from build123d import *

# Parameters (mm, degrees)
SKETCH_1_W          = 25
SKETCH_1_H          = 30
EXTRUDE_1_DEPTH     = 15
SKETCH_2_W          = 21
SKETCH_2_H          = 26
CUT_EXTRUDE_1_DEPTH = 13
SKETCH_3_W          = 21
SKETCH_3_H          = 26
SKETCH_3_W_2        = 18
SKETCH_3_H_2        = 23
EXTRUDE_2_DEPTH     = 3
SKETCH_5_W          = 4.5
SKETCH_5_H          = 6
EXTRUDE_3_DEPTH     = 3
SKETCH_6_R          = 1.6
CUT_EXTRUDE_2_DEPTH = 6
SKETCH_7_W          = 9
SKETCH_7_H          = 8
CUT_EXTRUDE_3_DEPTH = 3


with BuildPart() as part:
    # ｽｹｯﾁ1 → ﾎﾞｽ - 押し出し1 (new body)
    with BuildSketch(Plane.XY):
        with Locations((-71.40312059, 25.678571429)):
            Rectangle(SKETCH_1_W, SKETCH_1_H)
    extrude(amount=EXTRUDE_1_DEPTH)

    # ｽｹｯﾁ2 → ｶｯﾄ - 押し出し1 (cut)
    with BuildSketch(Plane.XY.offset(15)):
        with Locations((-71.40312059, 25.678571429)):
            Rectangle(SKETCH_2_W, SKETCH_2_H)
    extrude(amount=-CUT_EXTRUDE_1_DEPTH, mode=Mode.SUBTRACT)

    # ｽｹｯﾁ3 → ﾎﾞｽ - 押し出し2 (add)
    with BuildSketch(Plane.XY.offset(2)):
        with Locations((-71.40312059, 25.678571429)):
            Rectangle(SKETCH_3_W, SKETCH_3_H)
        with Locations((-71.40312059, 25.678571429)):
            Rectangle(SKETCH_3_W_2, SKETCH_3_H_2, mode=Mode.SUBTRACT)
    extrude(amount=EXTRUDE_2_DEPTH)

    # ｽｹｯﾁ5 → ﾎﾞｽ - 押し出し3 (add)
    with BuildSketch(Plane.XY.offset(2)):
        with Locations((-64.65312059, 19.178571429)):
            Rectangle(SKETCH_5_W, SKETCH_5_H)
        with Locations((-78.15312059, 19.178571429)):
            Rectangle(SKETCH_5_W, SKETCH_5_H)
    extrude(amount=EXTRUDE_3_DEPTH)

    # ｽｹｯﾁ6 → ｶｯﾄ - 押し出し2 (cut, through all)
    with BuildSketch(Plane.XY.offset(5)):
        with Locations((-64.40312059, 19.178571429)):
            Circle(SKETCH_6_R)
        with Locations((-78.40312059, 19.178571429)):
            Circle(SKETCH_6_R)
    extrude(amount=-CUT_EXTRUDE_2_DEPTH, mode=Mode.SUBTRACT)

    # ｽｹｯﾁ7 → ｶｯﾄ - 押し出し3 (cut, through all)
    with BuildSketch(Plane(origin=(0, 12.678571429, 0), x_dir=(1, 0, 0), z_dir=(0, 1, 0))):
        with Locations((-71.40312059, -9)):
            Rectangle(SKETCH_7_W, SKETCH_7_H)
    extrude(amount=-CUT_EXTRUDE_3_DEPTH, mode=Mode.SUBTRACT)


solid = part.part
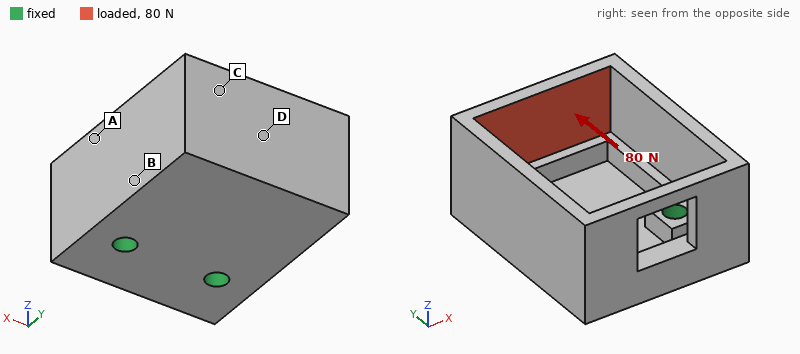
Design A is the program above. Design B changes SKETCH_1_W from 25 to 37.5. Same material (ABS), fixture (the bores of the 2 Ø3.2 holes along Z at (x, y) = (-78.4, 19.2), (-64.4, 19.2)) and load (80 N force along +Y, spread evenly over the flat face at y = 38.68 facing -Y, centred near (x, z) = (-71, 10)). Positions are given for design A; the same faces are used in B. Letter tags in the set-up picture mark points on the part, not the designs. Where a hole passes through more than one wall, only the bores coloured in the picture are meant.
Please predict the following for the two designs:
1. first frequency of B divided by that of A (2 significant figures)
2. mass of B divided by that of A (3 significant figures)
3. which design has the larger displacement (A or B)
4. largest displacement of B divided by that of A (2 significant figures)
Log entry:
0.73
2.25
A
0.76
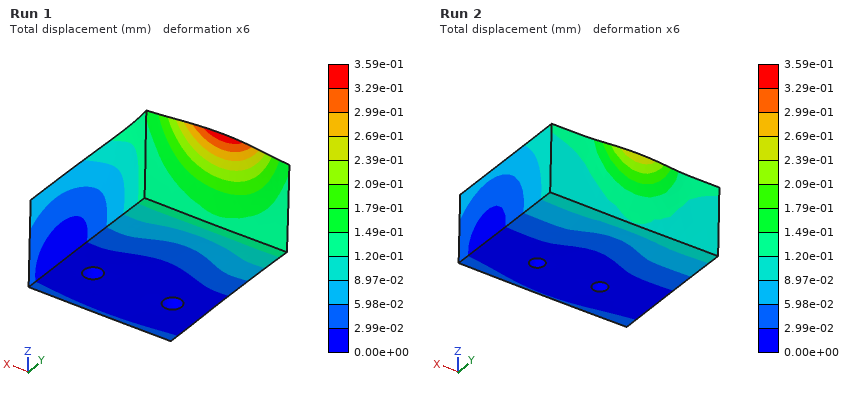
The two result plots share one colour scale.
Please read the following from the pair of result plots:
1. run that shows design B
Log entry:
Run 2
